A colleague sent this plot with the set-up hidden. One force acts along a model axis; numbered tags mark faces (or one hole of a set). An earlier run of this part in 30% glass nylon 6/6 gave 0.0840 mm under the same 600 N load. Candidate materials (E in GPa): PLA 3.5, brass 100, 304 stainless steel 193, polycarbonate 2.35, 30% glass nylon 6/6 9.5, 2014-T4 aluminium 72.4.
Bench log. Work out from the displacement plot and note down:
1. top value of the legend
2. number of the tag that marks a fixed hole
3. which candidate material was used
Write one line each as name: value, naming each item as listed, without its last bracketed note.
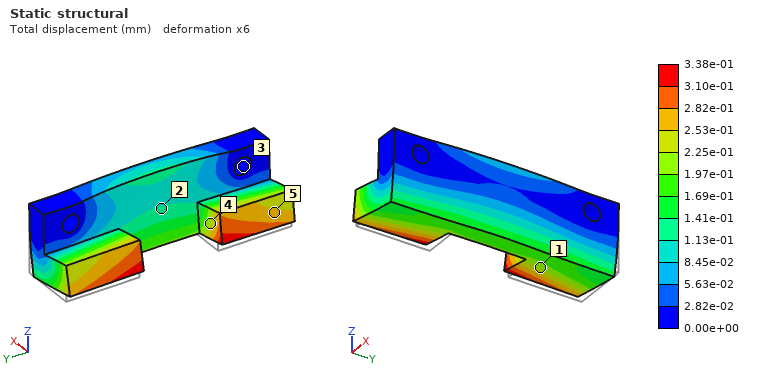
top value of the legend: 3.38e-01 mm
number of the tag that marks a fixed hole: 3
which candidate material was used: polycarbonate
